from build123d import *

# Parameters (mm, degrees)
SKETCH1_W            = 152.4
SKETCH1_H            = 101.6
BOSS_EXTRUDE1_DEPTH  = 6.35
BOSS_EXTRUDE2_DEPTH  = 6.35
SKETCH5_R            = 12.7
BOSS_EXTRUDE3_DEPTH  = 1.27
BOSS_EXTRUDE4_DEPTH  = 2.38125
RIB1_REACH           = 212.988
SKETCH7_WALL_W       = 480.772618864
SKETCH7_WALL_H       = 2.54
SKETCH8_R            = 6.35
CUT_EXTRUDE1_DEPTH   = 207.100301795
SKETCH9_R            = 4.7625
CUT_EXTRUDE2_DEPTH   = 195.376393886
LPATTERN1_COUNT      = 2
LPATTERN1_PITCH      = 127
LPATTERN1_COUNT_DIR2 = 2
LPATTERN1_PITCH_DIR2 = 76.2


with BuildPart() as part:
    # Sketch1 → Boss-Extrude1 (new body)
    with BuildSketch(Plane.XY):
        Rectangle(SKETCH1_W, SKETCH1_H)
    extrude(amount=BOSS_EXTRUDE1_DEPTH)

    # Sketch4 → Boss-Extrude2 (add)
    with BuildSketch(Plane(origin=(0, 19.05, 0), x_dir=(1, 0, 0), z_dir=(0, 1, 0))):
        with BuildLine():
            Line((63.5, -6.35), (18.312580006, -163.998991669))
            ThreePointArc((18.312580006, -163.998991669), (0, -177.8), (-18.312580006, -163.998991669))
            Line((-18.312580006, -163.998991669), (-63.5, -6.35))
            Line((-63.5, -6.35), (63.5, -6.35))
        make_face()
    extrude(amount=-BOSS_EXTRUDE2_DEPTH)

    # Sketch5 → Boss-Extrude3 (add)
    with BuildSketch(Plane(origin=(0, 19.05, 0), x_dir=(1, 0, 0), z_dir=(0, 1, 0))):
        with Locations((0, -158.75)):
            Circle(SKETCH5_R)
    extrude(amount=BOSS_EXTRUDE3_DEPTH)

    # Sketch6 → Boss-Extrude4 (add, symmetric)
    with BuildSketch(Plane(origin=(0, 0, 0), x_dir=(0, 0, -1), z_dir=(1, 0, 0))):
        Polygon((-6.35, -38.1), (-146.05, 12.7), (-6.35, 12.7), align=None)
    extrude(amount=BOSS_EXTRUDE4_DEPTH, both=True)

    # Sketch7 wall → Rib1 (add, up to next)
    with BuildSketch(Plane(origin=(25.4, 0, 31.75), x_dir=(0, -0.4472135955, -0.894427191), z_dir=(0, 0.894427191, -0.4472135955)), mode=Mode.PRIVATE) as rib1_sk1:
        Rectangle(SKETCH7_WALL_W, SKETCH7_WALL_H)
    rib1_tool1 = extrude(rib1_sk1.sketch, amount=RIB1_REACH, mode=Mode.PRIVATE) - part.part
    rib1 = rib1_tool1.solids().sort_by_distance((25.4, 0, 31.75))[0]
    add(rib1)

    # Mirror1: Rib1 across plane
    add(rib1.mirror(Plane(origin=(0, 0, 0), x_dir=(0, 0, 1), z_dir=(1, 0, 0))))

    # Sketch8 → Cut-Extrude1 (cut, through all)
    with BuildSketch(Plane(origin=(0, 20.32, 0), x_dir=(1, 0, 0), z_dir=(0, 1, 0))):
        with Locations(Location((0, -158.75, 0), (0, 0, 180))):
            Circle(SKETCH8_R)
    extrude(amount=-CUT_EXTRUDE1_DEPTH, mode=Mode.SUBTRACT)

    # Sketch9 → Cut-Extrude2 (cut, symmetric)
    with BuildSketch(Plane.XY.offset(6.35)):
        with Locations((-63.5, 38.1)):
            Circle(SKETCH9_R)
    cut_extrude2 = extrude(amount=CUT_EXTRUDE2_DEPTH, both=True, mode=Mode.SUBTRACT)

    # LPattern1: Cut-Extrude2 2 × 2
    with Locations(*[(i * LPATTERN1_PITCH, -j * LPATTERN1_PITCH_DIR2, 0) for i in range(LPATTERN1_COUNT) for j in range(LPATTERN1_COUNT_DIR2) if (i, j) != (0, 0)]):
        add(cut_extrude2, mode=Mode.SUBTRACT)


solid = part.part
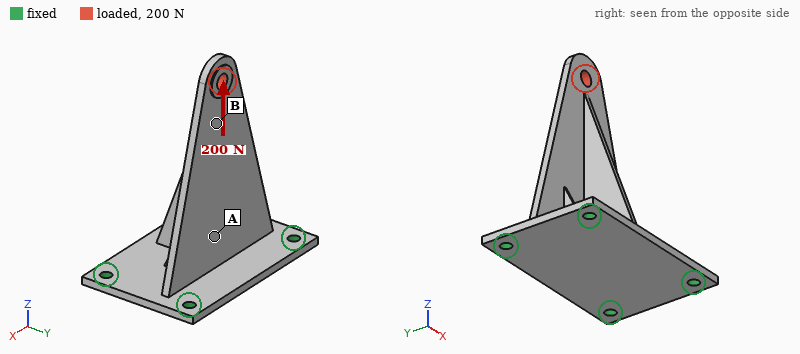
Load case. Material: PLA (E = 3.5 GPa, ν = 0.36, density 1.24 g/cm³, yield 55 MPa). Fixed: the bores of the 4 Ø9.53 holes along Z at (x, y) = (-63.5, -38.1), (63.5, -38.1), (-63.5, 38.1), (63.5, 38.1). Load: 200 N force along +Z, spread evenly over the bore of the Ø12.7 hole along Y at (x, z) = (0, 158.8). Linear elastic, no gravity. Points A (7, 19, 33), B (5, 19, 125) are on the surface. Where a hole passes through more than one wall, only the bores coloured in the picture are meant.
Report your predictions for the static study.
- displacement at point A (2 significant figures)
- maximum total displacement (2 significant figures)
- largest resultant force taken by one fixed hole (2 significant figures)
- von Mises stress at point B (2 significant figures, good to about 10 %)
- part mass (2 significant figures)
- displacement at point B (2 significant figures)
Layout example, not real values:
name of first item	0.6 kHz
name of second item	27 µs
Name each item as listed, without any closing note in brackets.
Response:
displacement at point A	0.049 mm
maximum total displacement	0.16 mm
largest resultant force taken by one fixed hole	82 N
von Mises stress at point B	0.87 MPa
part mass	250 g
displacement at point B	0.082 mm
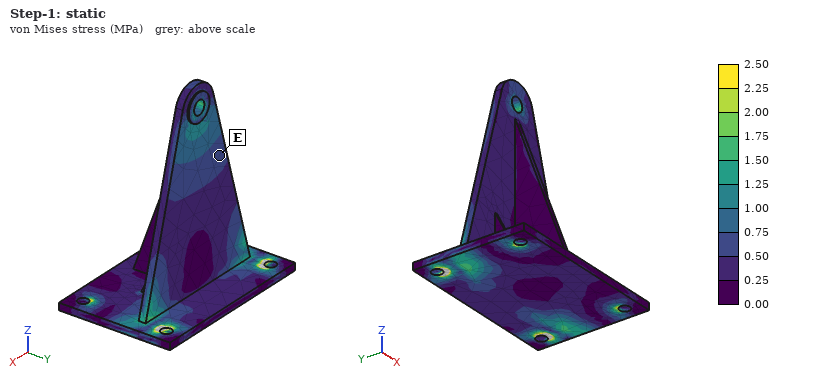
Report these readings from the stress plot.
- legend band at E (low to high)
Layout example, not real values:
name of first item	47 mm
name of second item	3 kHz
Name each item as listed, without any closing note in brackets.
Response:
legend band at E	0.50 to 0.75 MPa
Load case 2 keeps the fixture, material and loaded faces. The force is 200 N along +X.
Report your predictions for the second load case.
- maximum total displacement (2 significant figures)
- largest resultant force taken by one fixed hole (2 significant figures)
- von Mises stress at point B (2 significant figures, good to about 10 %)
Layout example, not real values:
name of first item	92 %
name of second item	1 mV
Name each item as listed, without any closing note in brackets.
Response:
maximum total displacement	0.54 mm
largest resultant force taken by one fixed hole	220 N
von Mises stress at point B	1.3 MPa
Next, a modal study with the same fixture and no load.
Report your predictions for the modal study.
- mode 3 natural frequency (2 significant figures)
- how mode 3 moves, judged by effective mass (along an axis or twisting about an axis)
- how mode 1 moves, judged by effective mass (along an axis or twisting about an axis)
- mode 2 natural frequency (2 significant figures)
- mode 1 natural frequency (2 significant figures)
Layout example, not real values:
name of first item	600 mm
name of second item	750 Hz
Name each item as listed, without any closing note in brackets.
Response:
mode 3 natural frequency	590 Hz
how mode 3 moves, judged by effective mass	along X
how mode 1 moves, judged by effective mass	along Y
mode 2 natural frequency	500 Hz
mode 1 natural frequency	190 Hz
